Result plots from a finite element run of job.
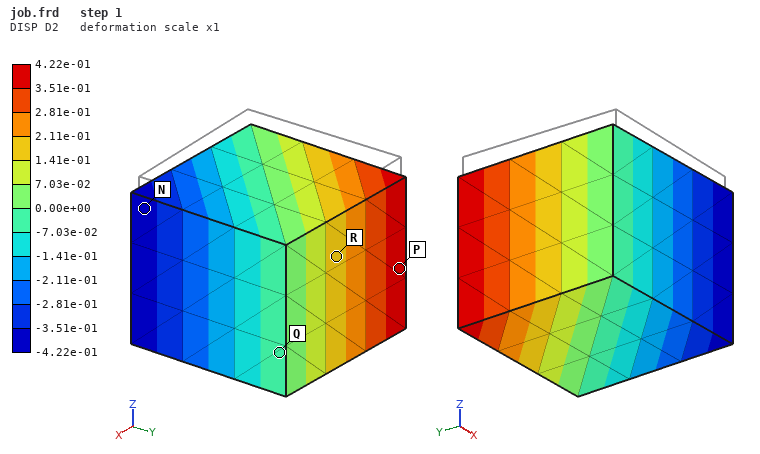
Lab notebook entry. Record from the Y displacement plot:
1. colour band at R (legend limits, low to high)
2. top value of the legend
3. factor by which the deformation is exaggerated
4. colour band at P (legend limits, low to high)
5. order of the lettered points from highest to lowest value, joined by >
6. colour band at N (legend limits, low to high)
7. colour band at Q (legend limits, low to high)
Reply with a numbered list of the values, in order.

1. 1.41e-01 to 2.11e-01
2. 4.22e-01
3. 1
4. 3.51e-01 to 4.22e-01
5. P > R > Q > N
6. -4.22e-01 to -3.51e-01
7. -7.03e-02 to 0.00e+00
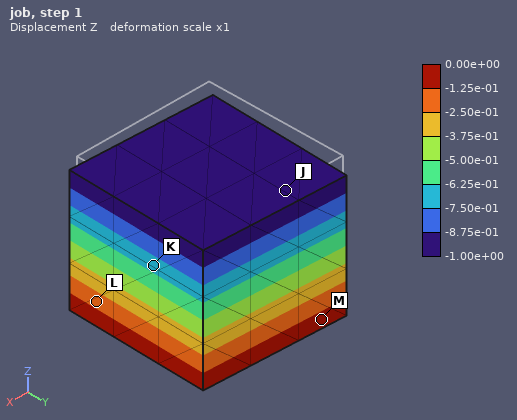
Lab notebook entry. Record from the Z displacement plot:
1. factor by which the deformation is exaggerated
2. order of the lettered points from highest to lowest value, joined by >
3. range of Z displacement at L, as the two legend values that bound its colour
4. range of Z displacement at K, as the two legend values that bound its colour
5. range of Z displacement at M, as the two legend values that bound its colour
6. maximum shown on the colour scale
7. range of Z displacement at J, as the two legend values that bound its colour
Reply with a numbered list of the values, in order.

1. 1
2. M > L > K > J
3. -2.50e-01 to -1.25e-01
4. -7.50e-01 to -6.25e-01
5. -1.25e-01 to 0.00e+00
6. 0.00e+00
7. -1.00e+00 to -8.75e-01
